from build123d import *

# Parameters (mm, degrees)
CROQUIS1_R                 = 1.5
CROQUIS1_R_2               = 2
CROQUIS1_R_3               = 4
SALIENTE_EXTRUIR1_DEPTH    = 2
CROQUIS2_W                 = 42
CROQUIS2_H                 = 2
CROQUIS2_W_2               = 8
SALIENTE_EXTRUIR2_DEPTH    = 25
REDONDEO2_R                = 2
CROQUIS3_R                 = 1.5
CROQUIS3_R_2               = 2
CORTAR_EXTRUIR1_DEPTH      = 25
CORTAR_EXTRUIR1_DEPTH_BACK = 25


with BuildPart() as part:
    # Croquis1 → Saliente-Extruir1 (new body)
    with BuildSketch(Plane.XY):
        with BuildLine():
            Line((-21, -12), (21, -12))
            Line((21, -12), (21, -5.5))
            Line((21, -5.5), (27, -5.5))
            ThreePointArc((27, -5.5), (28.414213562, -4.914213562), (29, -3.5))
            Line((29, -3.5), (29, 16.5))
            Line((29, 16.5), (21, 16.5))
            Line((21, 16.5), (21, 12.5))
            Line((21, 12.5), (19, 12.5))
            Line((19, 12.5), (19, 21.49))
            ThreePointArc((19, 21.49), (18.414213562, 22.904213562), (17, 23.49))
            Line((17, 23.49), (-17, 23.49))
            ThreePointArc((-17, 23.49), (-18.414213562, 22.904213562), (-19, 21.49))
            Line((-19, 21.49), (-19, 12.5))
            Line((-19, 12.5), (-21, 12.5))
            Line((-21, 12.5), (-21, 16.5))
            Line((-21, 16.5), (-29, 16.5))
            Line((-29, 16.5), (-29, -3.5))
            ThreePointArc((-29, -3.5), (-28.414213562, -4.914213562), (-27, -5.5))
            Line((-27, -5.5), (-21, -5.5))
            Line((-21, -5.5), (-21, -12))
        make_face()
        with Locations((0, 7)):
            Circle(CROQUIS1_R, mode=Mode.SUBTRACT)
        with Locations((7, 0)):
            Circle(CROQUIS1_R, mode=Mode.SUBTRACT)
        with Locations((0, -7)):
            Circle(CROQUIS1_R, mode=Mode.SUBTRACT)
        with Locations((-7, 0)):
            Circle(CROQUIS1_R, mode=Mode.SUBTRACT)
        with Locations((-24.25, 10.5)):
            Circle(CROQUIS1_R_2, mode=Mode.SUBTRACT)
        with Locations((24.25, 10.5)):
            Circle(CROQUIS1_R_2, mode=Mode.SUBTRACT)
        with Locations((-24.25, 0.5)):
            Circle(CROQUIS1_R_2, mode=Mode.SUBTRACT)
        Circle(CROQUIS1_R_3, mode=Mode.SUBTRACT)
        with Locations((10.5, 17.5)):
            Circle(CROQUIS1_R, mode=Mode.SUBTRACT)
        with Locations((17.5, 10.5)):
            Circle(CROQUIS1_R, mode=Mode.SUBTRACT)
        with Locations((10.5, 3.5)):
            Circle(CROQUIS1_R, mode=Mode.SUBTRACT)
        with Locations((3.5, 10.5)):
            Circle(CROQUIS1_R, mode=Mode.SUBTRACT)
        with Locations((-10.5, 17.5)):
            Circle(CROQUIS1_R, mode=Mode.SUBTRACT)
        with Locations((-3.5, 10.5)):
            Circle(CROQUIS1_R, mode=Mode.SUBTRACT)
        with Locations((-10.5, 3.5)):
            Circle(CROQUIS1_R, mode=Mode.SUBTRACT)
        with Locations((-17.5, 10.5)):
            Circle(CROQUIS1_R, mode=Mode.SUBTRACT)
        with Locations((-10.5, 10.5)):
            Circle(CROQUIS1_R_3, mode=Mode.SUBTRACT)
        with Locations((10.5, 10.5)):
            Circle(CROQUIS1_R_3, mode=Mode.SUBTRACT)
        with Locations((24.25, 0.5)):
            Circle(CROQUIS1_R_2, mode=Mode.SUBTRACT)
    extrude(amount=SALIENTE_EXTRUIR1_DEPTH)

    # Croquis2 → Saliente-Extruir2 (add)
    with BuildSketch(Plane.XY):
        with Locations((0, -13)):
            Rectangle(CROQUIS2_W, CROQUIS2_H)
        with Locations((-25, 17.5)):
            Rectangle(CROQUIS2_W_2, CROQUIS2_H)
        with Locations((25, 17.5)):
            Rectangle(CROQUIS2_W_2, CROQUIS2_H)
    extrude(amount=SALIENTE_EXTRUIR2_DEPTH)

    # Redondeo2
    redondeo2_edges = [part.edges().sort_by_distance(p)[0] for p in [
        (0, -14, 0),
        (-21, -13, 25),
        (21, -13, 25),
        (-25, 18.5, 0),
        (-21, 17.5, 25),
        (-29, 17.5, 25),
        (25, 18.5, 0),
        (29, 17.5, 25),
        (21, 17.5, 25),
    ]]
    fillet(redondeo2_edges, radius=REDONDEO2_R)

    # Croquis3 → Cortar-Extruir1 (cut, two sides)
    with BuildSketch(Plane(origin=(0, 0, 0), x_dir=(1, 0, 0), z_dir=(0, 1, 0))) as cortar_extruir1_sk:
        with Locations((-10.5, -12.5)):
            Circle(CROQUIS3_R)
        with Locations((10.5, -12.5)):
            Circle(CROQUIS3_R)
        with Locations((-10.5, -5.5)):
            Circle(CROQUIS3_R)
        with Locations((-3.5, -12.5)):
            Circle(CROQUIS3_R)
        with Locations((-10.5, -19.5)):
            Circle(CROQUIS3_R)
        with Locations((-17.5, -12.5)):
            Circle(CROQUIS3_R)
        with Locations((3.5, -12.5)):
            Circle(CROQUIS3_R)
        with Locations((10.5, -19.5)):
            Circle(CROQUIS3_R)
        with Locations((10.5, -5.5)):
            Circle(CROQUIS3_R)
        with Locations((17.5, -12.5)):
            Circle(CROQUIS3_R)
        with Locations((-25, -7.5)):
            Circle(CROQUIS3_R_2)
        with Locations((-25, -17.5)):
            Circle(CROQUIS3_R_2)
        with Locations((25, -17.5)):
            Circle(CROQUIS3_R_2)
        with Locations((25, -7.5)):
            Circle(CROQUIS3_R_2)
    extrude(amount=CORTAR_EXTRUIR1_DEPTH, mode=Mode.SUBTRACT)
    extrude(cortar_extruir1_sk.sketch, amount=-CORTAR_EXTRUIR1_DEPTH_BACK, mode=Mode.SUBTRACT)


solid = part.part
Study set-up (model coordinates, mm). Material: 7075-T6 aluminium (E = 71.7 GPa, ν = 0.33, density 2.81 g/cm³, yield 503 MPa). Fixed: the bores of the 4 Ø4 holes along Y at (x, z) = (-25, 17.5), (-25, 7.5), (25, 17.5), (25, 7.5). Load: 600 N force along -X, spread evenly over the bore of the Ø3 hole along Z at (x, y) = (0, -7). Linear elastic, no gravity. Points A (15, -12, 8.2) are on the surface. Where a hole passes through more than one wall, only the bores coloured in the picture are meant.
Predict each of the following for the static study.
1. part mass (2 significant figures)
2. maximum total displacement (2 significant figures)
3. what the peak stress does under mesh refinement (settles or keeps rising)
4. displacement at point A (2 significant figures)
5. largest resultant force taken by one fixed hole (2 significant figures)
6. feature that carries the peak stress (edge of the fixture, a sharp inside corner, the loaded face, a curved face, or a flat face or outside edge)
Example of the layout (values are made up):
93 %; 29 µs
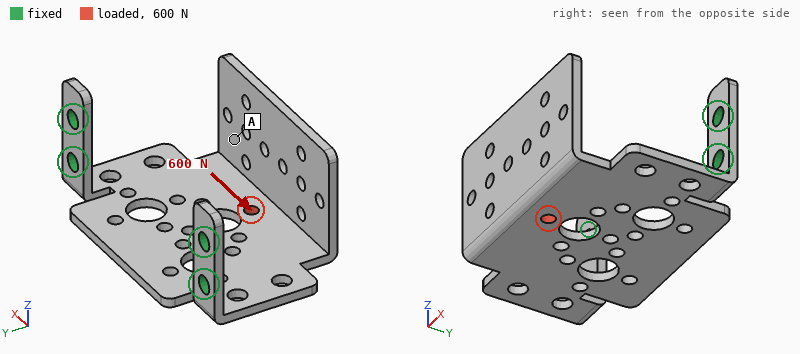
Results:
16 g; 0.17 mm; keeps rising; 0.11 mm; 430 N; edge of the fixture
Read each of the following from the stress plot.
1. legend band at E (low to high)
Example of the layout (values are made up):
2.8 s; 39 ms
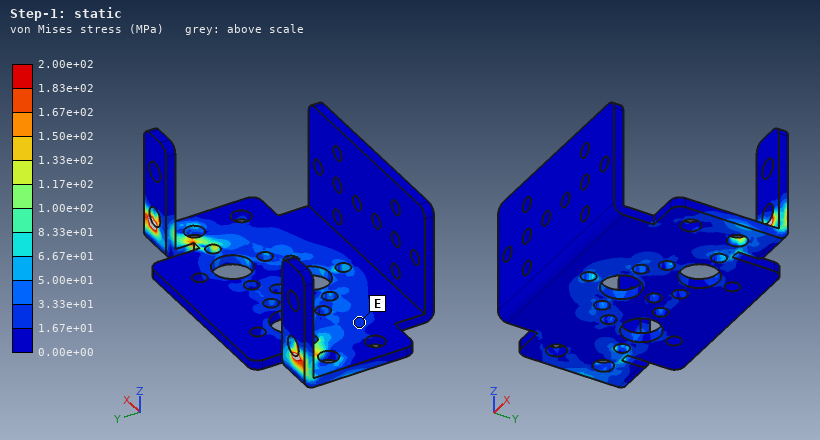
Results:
1.67e+01 to 3.33e+01 MPa
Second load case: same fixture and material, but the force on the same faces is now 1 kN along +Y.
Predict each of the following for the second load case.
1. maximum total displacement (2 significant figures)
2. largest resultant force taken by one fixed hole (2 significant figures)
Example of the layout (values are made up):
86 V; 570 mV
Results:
0.60 mm; 520 N
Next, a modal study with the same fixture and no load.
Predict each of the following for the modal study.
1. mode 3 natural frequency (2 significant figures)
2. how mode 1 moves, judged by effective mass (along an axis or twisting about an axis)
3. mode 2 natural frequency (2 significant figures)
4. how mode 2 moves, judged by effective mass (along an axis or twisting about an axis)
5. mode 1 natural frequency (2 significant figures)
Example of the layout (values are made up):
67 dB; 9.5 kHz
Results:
1700 Hz; along Z; 1300 Hz; along X; 400 Hz
